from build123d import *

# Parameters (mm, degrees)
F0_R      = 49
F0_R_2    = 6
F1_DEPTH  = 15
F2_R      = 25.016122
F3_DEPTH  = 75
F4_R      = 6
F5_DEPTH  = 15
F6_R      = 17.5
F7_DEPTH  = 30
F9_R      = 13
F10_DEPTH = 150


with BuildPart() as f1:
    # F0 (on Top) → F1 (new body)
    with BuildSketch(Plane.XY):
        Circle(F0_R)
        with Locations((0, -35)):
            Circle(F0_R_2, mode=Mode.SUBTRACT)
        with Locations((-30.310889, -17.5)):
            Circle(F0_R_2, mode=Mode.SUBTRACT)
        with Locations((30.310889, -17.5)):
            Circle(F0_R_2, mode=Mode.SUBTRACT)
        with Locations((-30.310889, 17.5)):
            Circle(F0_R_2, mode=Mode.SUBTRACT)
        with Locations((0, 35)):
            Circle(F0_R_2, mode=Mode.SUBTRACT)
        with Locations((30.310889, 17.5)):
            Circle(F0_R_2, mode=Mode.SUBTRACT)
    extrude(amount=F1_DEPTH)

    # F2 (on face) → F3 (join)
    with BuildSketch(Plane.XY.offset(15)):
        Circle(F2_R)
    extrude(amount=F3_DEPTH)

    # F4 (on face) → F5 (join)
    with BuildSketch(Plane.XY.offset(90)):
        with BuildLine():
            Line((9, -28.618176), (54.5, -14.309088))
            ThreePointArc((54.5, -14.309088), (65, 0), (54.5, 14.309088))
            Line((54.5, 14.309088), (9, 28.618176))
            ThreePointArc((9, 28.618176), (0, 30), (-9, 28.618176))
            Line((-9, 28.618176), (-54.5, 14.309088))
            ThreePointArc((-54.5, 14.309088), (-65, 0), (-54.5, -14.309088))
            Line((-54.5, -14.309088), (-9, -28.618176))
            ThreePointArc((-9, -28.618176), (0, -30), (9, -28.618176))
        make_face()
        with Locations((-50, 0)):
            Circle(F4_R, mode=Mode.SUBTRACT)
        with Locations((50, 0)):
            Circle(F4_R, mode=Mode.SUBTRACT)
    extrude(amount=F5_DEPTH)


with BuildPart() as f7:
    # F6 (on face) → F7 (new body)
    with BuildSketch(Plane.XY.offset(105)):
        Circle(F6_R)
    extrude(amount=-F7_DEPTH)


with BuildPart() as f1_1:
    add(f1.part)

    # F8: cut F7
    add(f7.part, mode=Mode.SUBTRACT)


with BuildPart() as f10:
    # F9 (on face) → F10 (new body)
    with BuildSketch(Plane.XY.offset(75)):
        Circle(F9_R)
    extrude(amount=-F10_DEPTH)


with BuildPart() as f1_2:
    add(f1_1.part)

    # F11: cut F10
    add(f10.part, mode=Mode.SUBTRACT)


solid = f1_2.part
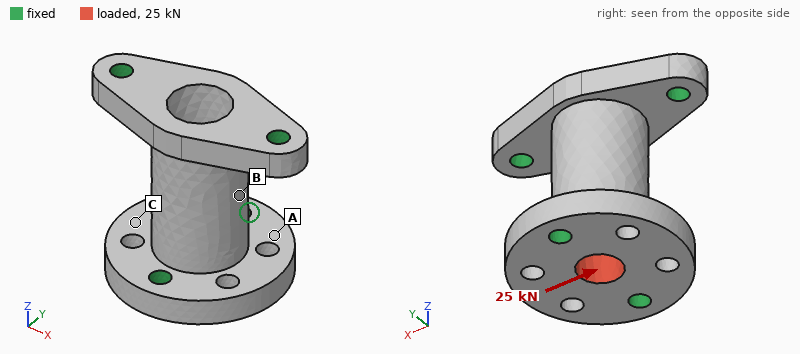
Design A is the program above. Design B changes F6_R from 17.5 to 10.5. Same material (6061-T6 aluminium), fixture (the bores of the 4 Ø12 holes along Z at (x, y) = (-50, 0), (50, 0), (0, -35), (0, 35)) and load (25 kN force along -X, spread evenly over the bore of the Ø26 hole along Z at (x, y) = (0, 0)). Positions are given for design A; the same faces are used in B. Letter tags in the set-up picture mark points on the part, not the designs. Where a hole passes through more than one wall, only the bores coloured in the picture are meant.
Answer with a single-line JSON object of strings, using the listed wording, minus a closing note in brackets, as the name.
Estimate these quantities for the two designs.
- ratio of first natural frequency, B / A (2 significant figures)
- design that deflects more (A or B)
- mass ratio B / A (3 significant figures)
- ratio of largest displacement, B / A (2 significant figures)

{"ratio of first natural frequency, B / A": "0.98", "design that deflects more": "A", "mass ratio B / A": "1.07", "ratio of largest displacement, B / A": "0.88"}
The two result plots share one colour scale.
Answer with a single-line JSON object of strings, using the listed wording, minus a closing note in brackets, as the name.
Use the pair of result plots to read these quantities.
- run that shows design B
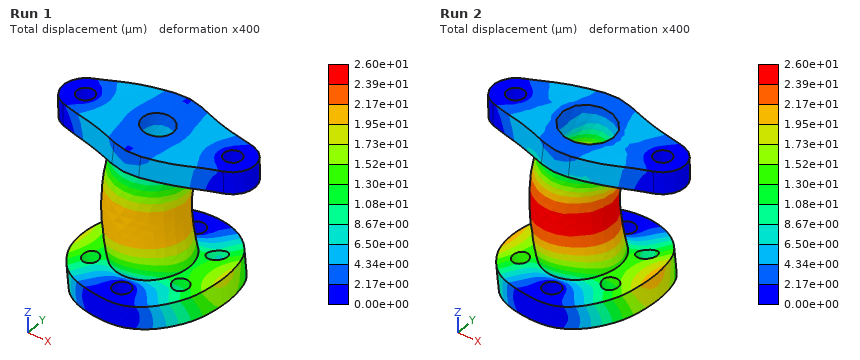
{"run that shows design B": "Run 1"}
